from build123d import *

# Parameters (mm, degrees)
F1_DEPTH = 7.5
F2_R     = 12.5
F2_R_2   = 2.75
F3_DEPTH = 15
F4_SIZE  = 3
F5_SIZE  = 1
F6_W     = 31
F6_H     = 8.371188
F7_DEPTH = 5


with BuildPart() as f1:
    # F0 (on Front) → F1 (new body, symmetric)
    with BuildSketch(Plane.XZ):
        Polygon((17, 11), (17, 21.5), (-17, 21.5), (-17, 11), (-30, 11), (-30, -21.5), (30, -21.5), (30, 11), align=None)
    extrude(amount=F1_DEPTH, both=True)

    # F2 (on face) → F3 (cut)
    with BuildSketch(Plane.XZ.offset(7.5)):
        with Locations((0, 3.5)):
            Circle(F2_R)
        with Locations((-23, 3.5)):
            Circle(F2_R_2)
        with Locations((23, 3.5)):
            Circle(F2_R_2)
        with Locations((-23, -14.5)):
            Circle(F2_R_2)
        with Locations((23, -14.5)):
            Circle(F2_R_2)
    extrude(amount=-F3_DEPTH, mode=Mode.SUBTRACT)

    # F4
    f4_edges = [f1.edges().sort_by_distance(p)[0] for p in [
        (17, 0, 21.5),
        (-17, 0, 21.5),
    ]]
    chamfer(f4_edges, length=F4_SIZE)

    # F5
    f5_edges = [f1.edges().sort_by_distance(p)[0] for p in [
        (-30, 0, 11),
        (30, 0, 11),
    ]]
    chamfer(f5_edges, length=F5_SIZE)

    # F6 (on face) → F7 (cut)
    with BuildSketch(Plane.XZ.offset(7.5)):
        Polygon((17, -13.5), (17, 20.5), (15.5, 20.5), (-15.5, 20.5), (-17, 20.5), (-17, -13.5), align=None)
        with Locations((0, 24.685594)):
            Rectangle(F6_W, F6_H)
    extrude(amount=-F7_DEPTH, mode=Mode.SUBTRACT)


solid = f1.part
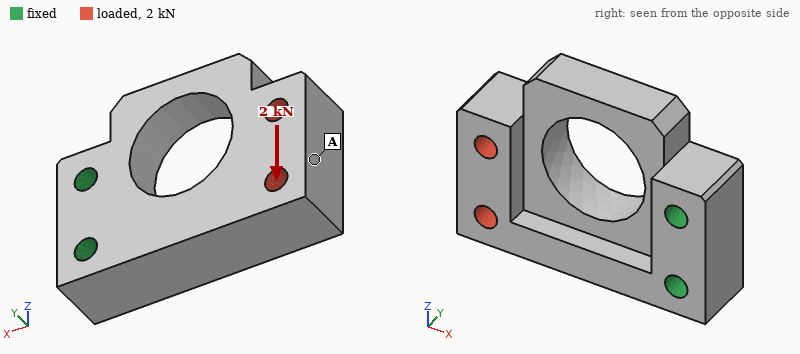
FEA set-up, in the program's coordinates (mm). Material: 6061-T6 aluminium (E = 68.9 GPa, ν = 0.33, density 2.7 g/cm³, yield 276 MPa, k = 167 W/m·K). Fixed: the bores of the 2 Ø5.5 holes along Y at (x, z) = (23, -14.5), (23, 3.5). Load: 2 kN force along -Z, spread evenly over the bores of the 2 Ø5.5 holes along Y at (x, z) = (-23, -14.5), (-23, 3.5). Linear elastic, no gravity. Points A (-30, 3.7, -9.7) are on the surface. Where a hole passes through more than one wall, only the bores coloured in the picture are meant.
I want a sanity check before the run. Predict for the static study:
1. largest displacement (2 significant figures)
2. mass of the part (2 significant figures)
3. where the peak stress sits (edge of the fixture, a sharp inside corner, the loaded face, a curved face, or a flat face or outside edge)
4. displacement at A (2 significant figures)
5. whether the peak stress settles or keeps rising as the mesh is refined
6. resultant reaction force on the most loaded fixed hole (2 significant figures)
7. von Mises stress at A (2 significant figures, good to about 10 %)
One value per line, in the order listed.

0.14 mm
60 g
a sharp inside corner
0.12 mm
keeps rising
4.1 kN
14 MPa
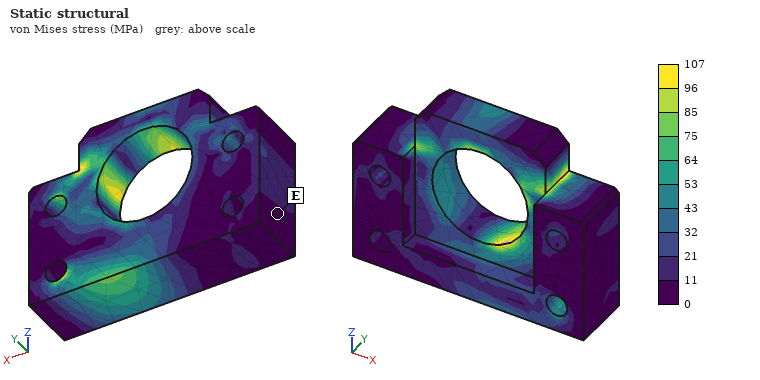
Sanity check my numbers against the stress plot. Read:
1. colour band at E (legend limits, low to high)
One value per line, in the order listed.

0 to 11 MPa
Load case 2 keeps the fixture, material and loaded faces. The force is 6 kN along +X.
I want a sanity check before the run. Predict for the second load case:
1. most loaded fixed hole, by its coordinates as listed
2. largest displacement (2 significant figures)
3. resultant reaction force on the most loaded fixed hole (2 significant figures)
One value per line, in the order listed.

(23, -14.5)
0.13 mm
3.2 kN
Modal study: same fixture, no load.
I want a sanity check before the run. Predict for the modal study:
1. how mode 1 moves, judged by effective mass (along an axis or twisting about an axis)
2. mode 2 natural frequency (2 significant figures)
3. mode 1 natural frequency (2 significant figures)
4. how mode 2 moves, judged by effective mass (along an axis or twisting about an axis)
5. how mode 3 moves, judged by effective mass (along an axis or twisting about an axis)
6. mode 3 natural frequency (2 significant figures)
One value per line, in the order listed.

along Y
4300 Hz
2900 Hz
along Z
twisting about X
6700 Hz
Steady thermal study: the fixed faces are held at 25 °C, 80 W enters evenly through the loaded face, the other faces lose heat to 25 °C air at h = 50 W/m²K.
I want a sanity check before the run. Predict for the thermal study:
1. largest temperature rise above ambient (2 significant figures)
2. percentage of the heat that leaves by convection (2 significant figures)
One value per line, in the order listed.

75 K
16 %
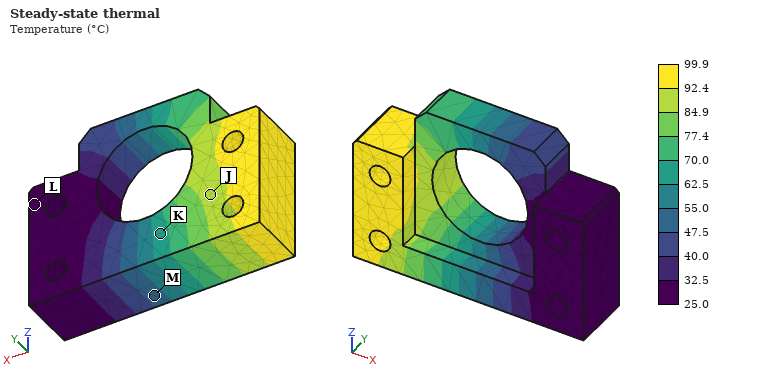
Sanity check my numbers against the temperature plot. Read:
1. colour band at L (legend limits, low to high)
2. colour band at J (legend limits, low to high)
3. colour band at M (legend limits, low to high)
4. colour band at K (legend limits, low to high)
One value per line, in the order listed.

25.0 to 32.5 °C
84.9 to 92.4 °C
47.5 to 55.0 °C
62.5 to 70.0 °C
